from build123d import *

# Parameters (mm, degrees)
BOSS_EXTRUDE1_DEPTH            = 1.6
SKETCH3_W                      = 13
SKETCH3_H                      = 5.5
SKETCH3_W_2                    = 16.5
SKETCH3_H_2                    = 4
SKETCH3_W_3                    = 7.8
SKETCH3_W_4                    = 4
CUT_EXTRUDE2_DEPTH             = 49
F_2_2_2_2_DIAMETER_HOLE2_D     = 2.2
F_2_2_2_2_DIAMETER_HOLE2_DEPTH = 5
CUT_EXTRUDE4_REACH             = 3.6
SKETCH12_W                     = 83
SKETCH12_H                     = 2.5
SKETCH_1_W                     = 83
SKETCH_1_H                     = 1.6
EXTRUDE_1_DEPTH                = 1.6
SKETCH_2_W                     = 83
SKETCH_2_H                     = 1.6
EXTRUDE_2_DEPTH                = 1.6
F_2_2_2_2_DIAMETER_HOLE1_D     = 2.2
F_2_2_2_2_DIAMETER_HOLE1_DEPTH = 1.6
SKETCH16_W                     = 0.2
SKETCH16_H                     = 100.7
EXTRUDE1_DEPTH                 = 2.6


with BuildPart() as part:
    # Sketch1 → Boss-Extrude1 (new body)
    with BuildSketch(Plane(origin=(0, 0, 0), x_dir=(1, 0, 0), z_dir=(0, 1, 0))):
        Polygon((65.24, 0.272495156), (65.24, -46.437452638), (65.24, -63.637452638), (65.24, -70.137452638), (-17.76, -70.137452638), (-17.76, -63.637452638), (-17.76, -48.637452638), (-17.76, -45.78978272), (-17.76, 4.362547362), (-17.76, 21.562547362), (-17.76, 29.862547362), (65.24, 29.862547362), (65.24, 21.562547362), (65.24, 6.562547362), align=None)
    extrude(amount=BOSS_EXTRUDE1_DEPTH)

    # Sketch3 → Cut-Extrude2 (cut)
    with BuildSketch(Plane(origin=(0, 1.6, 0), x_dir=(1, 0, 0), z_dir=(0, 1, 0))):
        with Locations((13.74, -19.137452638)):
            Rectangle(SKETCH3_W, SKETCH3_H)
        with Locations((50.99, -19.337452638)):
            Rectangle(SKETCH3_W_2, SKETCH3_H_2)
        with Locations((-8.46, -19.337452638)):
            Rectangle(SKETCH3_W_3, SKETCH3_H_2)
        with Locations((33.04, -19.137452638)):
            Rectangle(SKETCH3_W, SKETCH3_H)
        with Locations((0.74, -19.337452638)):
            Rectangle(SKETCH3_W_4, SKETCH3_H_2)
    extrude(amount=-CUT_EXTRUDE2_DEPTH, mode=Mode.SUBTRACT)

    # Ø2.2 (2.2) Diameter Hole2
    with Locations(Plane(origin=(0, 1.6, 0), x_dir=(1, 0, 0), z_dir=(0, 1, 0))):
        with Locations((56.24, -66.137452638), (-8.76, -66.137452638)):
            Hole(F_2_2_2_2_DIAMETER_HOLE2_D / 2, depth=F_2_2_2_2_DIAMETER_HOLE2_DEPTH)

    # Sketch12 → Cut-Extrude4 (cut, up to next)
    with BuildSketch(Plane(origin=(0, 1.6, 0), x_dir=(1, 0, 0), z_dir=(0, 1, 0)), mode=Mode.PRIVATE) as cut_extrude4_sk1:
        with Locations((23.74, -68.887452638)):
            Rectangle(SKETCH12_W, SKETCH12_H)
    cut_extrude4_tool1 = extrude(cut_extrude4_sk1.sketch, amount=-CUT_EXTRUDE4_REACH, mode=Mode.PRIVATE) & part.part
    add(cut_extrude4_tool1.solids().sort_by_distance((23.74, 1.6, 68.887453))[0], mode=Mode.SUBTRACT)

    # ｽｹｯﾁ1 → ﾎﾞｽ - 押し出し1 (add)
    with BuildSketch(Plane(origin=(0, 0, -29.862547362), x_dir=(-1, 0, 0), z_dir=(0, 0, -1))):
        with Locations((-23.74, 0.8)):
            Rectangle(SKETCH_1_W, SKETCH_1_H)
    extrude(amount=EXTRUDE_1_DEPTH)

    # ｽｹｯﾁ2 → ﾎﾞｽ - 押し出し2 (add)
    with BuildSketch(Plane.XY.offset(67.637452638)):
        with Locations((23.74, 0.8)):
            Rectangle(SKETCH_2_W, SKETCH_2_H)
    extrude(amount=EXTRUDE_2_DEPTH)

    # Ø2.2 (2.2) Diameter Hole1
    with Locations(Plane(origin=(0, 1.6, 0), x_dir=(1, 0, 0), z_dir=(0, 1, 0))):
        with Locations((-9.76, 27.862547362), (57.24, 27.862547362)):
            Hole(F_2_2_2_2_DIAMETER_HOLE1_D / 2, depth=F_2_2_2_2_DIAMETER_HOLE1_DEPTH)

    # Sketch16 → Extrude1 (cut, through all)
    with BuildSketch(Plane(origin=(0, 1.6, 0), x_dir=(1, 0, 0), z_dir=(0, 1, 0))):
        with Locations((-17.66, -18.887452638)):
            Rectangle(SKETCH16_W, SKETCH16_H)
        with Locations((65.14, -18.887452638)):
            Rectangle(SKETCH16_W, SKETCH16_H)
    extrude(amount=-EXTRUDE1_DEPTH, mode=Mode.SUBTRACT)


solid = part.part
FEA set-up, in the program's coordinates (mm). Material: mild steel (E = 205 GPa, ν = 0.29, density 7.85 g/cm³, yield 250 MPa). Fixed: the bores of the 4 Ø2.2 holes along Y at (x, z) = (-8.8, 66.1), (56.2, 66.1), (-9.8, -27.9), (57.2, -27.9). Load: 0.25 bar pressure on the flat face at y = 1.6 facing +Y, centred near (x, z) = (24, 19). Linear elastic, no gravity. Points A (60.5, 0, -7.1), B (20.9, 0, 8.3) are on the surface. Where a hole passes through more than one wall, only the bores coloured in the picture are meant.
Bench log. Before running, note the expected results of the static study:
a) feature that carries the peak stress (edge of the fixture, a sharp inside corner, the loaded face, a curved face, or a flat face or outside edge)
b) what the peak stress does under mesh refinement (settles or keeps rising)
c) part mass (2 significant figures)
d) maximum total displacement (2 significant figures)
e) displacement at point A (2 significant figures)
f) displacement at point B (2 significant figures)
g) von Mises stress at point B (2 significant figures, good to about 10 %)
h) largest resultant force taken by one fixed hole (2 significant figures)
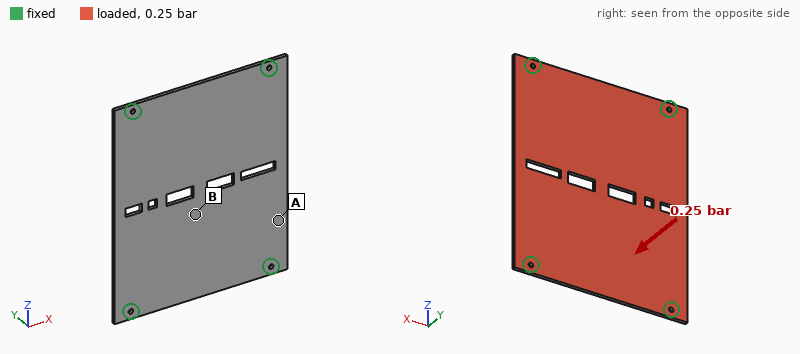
edge of the fixture
keeps rising
100 g
0.16 mm
0.061 mm
0.15 mm
19 MPa
51 N
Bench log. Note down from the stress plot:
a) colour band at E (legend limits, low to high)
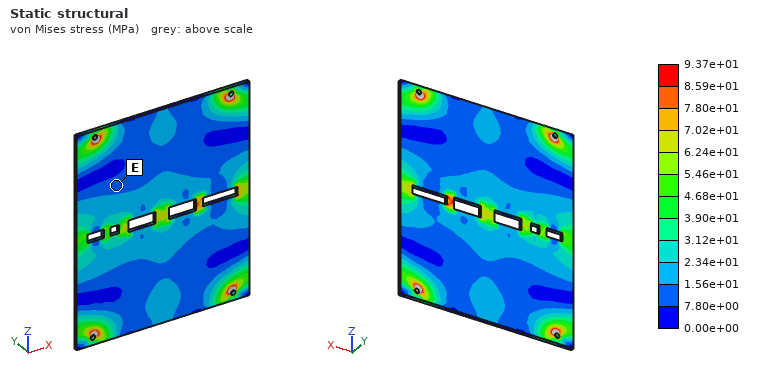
7.80e+00 to 1.56e+01 MPa
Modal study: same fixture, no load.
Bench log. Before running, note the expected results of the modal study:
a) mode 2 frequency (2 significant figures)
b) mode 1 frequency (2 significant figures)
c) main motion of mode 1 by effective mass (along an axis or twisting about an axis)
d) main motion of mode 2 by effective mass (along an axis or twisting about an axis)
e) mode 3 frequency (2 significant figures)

1100 Hz
680 Hz
along Y
twisting about Z
1600 Hz
